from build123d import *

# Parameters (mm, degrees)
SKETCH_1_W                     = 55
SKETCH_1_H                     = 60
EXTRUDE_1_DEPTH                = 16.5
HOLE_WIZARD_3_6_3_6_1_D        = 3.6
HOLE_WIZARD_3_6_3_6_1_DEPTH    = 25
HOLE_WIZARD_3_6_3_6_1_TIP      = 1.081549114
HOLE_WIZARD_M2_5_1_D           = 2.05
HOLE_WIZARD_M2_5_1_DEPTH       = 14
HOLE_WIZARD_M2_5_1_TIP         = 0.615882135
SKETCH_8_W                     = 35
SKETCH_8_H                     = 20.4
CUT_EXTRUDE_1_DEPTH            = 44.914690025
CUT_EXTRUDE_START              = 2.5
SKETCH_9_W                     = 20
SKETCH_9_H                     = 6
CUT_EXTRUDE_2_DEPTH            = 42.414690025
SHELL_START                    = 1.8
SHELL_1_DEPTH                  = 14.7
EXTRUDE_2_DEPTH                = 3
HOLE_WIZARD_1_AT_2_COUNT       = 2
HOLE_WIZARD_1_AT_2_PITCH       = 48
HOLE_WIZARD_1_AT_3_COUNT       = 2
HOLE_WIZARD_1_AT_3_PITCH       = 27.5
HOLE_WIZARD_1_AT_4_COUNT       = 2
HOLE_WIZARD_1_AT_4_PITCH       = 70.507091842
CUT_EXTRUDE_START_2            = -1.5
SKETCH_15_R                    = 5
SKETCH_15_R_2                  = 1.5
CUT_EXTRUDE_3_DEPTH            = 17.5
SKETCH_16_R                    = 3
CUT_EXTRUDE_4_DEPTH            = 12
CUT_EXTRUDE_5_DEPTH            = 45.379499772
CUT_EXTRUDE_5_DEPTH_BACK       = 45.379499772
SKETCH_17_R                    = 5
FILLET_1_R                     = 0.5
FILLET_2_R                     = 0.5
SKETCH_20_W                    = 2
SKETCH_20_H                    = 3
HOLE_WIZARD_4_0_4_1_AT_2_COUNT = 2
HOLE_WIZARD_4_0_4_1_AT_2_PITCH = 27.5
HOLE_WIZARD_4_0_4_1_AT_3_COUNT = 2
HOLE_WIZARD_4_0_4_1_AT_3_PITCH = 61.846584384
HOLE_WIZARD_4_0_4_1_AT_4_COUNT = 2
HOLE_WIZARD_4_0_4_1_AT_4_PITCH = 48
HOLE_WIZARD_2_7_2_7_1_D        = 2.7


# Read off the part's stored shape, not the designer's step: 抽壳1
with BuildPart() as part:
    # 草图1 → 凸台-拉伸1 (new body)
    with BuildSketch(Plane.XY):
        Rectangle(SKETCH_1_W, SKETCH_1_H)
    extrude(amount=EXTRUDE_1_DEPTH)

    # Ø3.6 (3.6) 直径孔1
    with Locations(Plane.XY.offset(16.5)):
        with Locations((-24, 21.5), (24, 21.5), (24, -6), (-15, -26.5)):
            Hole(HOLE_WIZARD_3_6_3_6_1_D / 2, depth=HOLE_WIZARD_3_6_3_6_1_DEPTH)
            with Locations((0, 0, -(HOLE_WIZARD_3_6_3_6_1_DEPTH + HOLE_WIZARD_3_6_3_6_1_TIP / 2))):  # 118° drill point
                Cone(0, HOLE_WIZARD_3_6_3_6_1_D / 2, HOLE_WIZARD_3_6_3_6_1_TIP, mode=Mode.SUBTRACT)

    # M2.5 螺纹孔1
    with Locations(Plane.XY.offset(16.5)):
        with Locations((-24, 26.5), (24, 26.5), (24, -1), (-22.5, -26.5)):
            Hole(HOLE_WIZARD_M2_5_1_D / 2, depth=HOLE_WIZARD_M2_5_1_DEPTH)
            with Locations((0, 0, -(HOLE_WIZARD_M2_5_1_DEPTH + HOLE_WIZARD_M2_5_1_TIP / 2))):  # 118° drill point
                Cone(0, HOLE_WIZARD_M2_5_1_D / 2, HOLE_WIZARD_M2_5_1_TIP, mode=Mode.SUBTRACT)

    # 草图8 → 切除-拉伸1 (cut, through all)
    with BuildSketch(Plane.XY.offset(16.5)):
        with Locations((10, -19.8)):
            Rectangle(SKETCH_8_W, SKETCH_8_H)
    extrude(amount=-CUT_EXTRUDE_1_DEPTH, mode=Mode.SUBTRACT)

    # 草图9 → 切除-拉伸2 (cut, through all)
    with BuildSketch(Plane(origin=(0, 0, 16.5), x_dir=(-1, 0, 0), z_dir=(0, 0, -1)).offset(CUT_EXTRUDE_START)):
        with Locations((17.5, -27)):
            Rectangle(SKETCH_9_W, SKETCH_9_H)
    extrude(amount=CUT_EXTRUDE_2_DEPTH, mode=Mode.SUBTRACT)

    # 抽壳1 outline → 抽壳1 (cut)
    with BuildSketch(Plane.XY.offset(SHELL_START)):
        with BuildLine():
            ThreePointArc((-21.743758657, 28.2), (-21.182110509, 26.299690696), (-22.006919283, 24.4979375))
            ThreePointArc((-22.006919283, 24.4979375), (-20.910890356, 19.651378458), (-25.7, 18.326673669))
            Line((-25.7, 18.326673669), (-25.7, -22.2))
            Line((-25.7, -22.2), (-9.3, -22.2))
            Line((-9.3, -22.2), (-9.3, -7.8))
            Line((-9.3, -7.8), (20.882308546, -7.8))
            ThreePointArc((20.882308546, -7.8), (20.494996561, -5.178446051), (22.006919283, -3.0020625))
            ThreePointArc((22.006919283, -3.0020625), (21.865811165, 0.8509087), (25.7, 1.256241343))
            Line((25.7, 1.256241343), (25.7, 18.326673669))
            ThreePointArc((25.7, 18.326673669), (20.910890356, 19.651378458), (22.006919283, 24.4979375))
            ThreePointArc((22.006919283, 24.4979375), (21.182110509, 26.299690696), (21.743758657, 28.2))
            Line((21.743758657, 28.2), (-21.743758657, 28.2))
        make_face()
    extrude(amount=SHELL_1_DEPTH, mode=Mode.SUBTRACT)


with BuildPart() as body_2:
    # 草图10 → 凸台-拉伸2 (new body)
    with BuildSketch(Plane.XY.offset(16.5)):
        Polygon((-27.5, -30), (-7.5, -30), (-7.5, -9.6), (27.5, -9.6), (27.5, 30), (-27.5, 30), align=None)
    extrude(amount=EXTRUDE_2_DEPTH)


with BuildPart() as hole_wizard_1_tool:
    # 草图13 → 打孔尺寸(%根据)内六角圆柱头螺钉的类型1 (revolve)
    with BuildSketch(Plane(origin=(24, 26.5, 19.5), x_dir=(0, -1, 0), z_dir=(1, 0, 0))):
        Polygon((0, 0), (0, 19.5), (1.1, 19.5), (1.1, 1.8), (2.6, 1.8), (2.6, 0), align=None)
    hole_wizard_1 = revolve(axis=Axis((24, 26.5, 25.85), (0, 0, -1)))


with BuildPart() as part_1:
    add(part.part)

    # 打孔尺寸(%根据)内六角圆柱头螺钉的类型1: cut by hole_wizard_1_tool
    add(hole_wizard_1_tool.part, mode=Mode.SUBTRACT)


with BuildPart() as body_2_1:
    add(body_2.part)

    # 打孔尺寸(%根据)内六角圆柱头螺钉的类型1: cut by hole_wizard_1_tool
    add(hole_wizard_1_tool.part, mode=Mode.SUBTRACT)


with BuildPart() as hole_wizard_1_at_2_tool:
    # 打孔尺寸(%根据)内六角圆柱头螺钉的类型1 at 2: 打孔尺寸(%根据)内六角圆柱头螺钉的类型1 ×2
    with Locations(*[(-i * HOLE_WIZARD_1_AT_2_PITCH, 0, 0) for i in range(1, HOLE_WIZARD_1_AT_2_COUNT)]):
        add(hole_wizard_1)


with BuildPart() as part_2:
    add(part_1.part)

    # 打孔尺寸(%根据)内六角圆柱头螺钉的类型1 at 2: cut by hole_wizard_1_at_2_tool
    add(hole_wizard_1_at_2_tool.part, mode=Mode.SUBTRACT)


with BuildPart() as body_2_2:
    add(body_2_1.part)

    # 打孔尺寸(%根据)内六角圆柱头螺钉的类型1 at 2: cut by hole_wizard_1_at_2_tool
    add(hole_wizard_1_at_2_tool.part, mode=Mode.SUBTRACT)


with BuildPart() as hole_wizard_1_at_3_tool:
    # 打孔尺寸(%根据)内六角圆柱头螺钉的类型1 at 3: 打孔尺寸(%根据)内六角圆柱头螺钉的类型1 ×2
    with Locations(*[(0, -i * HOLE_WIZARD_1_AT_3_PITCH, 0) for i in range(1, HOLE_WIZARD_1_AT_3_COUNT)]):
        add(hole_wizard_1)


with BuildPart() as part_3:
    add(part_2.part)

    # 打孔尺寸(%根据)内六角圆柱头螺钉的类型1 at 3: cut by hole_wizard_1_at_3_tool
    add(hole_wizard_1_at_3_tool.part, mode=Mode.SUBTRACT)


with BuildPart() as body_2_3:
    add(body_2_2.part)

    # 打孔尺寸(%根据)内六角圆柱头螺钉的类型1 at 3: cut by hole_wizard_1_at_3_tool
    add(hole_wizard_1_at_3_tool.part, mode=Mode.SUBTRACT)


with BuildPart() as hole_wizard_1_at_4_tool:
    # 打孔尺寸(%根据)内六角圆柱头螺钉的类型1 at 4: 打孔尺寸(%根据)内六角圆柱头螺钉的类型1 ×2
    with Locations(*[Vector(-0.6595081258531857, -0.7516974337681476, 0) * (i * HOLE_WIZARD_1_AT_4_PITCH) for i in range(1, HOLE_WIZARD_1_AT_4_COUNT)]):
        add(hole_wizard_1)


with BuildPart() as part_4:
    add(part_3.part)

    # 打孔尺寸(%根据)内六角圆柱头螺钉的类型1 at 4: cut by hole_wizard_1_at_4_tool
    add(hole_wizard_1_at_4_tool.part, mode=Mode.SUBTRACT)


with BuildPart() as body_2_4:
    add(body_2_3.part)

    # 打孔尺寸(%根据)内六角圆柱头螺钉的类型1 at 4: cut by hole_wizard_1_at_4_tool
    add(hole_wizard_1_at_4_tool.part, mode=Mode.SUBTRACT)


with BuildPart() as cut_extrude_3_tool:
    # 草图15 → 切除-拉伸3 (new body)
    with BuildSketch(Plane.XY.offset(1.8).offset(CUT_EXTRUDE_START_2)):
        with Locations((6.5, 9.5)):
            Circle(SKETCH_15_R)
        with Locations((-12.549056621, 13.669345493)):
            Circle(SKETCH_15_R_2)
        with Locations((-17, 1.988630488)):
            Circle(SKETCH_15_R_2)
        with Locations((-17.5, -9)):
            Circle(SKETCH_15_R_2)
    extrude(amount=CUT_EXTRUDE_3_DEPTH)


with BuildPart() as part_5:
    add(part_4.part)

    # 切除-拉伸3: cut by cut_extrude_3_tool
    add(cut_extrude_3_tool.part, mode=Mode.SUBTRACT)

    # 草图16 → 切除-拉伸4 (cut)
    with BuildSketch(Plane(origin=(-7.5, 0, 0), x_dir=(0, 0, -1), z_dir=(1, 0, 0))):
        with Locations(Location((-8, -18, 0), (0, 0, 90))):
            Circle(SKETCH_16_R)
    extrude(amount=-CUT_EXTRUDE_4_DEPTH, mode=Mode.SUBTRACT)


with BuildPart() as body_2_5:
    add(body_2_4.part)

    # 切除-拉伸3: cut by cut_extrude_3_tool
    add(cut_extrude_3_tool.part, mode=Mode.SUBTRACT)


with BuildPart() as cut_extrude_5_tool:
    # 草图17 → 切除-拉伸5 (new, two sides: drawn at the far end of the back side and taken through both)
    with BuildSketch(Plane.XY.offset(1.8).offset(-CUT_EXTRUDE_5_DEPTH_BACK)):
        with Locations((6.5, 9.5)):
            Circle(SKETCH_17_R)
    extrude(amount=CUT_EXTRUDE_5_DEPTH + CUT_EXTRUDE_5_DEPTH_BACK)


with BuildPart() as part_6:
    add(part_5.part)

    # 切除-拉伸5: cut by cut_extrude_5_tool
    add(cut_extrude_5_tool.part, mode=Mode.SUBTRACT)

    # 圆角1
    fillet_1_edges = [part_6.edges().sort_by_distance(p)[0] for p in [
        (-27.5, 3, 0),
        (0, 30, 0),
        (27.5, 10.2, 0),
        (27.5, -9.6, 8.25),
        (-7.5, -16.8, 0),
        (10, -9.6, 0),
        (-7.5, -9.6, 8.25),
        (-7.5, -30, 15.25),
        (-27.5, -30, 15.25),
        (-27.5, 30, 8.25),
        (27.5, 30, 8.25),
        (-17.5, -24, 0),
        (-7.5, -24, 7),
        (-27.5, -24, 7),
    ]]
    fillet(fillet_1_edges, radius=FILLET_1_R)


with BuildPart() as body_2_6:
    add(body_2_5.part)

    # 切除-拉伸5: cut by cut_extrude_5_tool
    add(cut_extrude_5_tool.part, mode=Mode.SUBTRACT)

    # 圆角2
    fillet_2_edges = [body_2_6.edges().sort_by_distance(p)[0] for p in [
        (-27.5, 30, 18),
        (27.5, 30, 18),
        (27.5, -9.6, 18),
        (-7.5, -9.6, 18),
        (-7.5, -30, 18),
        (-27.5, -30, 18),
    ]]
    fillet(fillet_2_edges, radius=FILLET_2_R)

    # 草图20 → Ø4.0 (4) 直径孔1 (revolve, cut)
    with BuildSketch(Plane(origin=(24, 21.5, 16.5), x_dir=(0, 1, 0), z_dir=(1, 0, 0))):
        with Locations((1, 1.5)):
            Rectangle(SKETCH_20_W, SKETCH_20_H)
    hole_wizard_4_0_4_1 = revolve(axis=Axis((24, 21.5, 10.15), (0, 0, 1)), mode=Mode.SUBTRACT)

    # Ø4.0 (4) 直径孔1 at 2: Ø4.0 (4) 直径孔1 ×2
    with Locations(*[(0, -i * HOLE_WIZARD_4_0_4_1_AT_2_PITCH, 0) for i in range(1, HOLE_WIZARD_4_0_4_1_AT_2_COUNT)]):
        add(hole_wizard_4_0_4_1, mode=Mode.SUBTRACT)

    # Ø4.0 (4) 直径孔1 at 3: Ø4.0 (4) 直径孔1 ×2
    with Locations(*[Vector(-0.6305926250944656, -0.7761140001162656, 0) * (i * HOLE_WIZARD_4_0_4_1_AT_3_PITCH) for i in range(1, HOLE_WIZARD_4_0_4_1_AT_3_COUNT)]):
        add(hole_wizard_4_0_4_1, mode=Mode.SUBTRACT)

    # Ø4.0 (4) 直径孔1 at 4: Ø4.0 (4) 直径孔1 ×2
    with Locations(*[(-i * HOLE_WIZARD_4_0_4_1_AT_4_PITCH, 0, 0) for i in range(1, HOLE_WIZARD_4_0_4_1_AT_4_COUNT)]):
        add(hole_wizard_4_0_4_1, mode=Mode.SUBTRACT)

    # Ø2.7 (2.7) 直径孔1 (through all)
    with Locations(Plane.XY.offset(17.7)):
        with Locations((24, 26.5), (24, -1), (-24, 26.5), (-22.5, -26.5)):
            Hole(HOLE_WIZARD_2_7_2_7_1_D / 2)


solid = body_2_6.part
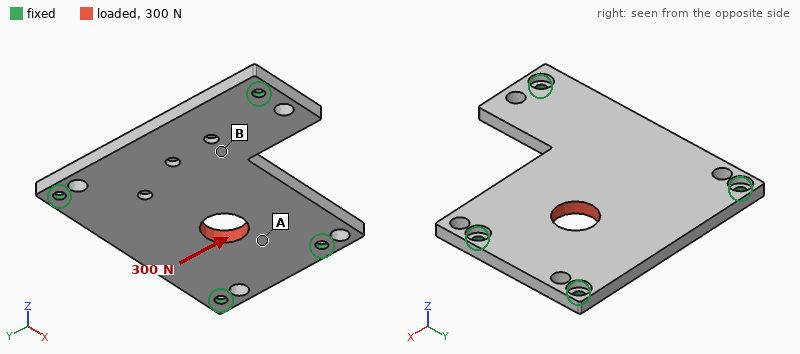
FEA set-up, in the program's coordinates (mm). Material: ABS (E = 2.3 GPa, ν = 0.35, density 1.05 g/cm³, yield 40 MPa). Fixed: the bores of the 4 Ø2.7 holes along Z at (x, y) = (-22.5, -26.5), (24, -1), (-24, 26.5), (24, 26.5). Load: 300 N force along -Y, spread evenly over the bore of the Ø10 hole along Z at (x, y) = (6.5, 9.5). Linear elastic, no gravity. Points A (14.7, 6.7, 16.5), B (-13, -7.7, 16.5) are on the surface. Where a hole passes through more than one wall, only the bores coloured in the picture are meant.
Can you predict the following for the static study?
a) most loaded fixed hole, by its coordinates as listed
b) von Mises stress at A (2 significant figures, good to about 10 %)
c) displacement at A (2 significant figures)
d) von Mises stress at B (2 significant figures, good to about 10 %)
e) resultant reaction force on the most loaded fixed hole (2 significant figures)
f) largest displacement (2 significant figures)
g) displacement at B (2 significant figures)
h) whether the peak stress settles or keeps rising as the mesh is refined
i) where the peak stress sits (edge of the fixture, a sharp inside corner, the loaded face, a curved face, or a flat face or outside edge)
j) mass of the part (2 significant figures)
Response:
(24, -1)
3.9 MPa
41 µm
1.8 MPa
110 N
63 µm
37 µm
keeps rising
edge of the fixture
7.5 g
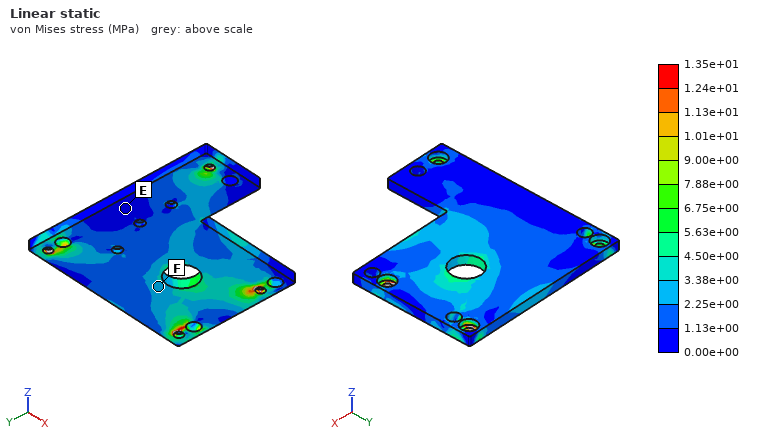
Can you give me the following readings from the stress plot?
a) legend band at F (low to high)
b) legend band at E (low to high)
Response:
2.25e+00 to 3.38e+00 MPa
0.00e+00 to 1.13e+00 MPa
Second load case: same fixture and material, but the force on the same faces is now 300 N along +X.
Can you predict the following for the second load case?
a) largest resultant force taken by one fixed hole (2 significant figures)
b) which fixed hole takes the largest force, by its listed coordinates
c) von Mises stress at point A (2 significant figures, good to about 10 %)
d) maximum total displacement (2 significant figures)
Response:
120 N
(24, -1)
3.7 MPa
68 µm
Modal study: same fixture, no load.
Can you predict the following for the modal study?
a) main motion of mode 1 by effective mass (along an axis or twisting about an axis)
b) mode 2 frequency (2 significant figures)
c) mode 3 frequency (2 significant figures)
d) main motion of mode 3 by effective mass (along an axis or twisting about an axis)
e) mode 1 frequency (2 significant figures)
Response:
along Z
1600 Hz
1900 Hz
twisting about X
1000 Hz
